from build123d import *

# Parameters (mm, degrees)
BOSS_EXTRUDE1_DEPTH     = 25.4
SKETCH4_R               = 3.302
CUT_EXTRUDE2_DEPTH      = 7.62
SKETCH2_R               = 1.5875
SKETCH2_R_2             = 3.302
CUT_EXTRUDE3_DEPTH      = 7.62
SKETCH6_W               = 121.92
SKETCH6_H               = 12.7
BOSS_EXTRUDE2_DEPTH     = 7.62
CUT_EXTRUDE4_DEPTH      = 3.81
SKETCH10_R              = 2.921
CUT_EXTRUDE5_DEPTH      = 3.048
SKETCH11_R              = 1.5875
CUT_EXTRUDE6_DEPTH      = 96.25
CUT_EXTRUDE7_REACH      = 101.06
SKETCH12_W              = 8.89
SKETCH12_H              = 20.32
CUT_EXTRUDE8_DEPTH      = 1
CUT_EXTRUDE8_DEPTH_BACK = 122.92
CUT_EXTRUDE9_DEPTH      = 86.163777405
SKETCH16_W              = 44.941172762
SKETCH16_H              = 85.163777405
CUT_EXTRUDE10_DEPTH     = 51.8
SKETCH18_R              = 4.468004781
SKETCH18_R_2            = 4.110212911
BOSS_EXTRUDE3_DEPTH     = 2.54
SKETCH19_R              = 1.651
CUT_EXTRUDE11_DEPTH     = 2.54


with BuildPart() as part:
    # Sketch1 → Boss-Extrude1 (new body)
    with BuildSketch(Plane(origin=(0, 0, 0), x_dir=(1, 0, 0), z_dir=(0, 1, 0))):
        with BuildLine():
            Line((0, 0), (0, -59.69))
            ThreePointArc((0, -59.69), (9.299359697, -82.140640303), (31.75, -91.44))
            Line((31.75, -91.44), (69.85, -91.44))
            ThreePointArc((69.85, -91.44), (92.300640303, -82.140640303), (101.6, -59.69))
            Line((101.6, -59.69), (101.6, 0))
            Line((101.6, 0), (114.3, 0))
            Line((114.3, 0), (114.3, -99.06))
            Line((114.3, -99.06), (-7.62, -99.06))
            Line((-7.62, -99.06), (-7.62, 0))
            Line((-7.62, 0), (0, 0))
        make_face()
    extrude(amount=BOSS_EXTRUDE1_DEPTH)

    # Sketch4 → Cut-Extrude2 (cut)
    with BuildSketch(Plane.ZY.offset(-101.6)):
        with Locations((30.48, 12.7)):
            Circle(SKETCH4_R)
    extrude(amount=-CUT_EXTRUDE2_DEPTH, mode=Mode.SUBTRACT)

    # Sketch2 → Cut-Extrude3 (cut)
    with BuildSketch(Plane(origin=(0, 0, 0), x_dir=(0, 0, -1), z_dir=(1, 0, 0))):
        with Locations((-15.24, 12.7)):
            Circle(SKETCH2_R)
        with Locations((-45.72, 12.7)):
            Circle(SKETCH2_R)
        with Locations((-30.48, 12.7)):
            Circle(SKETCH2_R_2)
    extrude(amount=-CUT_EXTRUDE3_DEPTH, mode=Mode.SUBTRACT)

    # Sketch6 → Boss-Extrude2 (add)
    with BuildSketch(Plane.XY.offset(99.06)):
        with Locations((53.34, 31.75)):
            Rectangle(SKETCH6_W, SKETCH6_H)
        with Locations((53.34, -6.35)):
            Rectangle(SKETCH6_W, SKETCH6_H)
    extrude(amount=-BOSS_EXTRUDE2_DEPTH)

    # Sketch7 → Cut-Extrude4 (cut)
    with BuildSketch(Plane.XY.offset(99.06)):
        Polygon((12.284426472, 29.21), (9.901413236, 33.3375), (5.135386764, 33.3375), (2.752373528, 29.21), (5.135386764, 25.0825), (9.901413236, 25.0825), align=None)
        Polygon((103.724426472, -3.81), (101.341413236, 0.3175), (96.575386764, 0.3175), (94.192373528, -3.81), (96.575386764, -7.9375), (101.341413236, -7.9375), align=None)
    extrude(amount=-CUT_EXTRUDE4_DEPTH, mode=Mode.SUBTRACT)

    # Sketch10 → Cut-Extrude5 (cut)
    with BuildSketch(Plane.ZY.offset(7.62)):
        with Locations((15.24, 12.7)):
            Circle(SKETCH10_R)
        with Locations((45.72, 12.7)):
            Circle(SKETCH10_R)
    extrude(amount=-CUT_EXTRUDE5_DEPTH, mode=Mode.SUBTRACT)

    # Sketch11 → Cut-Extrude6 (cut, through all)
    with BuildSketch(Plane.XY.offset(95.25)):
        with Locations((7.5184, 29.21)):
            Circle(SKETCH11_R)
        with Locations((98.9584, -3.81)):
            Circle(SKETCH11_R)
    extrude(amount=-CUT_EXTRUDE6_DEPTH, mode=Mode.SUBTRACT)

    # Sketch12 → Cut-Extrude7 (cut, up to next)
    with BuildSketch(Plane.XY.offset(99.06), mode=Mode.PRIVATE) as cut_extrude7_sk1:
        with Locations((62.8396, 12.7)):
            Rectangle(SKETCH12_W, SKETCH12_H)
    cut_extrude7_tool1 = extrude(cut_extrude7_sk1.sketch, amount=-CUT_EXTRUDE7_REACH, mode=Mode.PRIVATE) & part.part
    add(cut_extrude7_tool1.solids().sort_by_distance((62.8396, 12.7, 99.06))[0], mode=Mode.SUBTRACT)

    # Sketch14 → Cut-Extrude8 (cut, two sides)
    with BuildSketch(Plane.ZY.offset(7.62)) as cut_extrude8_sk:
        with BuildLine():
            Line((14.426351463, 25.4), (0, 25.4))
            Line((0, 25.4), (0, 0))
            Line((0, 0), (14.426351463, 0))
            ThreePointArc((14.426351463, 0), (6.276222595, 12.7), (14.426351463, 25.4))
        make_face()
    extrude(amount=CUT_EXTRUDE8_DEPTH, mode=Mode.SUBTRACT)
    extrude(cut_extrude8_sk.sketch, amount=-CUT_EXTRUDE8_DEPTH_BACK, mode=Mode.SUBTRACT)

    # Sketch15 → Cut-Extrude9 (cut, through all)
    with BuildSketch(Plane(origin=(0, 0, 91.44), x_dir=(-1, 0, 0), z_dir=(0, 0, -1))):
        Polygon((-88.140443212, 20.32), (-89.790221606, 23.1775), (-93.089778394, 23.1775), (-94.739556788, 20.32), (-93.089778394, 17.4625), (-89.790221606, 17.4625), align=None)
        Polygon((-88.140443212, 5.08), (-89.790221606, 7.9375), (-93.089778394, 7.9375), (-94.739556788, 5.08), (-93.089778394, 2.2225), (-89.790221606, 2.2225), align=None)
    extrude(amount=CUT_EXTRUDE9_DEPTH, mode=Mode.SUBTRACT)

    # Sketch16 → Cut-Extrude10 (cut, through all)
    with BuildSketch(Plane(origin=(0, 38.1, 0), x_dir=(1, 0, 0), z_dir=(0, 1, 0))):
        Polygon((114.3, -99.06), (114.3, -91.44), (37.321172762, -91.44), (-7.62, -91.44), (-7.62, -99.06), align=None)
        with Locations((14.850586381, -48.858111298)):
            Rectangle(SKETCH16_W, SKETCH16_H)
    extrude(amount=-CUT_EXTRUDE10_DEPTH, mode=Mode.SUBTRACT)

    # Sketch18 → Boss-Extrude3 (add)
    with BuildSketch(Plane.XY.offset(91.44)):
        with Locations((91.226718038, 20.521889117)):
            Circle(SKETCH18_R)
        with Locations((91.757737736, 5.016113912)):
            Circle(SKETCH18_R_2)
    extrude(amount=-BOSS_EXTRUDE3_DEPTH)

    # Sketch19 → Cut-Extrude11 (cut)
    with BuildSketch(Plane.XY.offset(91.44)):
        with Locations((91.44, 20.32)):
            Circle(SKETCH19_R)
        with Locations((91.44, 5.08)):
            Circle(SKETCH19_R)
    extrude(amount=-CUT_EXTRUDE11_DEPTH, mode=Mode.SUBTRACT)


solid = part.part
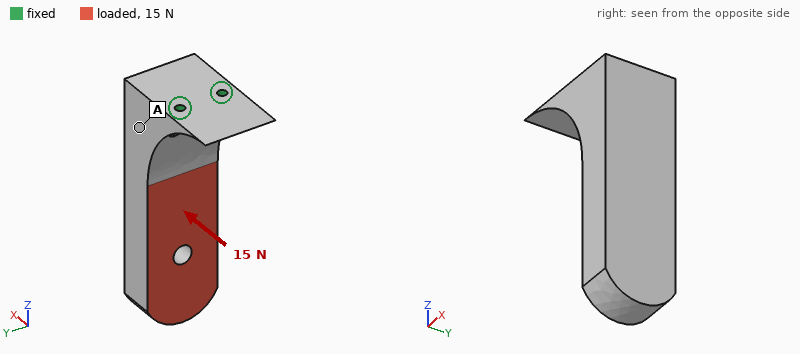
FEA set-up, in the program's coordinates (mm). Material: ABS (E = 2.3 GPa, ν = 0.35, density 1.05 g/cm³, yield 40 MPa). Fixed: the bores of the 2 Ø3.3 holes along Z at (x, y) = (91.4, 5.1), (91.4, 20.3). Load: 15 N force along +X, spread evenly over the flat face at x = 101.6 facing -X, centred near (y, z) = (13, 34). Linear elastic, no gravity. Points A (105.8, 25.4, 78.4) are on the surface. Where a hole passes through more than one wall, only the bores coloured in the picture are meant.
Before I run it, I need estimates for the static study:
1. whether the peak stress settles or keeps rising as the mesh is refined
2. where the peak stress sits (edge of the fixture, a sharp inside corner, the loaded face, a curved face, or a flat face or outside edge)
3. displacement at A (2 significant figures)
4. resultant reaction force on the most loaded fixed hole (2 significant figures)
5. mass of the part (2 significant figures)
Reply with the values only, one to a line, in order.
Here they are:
keeps rising
edge of the fixture
0.19 mm
7.9 N
33 g
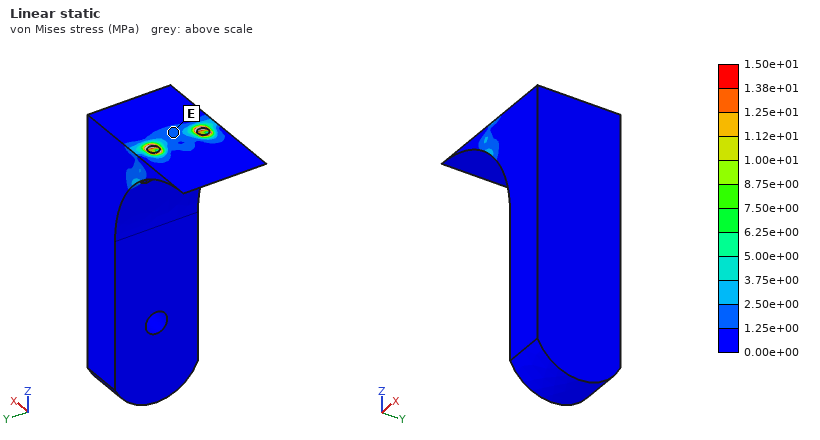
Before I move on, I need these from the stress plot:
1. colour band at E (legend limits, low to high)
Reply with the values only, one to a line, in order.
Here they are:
1.25e+00 to 2.50e+00 MPa
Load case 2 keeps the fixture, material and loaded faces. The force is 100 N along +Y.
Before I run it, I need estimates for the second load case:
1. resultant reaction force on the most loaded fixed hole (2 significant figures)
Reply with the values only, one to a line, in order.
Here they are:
340 N
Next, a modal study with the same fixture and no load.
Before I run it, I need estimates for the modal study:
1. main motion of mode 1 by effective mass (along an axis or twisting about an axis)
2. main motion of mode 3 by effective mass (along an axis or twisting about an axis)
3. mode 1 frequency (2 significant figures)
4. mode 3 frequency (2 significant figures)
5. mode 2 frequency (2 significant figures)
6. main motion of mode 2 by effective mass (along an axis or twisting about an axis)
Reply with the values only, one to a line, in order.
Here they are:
along X
along Z
170 Hz
1400 Hz
450 Hz
along Y
